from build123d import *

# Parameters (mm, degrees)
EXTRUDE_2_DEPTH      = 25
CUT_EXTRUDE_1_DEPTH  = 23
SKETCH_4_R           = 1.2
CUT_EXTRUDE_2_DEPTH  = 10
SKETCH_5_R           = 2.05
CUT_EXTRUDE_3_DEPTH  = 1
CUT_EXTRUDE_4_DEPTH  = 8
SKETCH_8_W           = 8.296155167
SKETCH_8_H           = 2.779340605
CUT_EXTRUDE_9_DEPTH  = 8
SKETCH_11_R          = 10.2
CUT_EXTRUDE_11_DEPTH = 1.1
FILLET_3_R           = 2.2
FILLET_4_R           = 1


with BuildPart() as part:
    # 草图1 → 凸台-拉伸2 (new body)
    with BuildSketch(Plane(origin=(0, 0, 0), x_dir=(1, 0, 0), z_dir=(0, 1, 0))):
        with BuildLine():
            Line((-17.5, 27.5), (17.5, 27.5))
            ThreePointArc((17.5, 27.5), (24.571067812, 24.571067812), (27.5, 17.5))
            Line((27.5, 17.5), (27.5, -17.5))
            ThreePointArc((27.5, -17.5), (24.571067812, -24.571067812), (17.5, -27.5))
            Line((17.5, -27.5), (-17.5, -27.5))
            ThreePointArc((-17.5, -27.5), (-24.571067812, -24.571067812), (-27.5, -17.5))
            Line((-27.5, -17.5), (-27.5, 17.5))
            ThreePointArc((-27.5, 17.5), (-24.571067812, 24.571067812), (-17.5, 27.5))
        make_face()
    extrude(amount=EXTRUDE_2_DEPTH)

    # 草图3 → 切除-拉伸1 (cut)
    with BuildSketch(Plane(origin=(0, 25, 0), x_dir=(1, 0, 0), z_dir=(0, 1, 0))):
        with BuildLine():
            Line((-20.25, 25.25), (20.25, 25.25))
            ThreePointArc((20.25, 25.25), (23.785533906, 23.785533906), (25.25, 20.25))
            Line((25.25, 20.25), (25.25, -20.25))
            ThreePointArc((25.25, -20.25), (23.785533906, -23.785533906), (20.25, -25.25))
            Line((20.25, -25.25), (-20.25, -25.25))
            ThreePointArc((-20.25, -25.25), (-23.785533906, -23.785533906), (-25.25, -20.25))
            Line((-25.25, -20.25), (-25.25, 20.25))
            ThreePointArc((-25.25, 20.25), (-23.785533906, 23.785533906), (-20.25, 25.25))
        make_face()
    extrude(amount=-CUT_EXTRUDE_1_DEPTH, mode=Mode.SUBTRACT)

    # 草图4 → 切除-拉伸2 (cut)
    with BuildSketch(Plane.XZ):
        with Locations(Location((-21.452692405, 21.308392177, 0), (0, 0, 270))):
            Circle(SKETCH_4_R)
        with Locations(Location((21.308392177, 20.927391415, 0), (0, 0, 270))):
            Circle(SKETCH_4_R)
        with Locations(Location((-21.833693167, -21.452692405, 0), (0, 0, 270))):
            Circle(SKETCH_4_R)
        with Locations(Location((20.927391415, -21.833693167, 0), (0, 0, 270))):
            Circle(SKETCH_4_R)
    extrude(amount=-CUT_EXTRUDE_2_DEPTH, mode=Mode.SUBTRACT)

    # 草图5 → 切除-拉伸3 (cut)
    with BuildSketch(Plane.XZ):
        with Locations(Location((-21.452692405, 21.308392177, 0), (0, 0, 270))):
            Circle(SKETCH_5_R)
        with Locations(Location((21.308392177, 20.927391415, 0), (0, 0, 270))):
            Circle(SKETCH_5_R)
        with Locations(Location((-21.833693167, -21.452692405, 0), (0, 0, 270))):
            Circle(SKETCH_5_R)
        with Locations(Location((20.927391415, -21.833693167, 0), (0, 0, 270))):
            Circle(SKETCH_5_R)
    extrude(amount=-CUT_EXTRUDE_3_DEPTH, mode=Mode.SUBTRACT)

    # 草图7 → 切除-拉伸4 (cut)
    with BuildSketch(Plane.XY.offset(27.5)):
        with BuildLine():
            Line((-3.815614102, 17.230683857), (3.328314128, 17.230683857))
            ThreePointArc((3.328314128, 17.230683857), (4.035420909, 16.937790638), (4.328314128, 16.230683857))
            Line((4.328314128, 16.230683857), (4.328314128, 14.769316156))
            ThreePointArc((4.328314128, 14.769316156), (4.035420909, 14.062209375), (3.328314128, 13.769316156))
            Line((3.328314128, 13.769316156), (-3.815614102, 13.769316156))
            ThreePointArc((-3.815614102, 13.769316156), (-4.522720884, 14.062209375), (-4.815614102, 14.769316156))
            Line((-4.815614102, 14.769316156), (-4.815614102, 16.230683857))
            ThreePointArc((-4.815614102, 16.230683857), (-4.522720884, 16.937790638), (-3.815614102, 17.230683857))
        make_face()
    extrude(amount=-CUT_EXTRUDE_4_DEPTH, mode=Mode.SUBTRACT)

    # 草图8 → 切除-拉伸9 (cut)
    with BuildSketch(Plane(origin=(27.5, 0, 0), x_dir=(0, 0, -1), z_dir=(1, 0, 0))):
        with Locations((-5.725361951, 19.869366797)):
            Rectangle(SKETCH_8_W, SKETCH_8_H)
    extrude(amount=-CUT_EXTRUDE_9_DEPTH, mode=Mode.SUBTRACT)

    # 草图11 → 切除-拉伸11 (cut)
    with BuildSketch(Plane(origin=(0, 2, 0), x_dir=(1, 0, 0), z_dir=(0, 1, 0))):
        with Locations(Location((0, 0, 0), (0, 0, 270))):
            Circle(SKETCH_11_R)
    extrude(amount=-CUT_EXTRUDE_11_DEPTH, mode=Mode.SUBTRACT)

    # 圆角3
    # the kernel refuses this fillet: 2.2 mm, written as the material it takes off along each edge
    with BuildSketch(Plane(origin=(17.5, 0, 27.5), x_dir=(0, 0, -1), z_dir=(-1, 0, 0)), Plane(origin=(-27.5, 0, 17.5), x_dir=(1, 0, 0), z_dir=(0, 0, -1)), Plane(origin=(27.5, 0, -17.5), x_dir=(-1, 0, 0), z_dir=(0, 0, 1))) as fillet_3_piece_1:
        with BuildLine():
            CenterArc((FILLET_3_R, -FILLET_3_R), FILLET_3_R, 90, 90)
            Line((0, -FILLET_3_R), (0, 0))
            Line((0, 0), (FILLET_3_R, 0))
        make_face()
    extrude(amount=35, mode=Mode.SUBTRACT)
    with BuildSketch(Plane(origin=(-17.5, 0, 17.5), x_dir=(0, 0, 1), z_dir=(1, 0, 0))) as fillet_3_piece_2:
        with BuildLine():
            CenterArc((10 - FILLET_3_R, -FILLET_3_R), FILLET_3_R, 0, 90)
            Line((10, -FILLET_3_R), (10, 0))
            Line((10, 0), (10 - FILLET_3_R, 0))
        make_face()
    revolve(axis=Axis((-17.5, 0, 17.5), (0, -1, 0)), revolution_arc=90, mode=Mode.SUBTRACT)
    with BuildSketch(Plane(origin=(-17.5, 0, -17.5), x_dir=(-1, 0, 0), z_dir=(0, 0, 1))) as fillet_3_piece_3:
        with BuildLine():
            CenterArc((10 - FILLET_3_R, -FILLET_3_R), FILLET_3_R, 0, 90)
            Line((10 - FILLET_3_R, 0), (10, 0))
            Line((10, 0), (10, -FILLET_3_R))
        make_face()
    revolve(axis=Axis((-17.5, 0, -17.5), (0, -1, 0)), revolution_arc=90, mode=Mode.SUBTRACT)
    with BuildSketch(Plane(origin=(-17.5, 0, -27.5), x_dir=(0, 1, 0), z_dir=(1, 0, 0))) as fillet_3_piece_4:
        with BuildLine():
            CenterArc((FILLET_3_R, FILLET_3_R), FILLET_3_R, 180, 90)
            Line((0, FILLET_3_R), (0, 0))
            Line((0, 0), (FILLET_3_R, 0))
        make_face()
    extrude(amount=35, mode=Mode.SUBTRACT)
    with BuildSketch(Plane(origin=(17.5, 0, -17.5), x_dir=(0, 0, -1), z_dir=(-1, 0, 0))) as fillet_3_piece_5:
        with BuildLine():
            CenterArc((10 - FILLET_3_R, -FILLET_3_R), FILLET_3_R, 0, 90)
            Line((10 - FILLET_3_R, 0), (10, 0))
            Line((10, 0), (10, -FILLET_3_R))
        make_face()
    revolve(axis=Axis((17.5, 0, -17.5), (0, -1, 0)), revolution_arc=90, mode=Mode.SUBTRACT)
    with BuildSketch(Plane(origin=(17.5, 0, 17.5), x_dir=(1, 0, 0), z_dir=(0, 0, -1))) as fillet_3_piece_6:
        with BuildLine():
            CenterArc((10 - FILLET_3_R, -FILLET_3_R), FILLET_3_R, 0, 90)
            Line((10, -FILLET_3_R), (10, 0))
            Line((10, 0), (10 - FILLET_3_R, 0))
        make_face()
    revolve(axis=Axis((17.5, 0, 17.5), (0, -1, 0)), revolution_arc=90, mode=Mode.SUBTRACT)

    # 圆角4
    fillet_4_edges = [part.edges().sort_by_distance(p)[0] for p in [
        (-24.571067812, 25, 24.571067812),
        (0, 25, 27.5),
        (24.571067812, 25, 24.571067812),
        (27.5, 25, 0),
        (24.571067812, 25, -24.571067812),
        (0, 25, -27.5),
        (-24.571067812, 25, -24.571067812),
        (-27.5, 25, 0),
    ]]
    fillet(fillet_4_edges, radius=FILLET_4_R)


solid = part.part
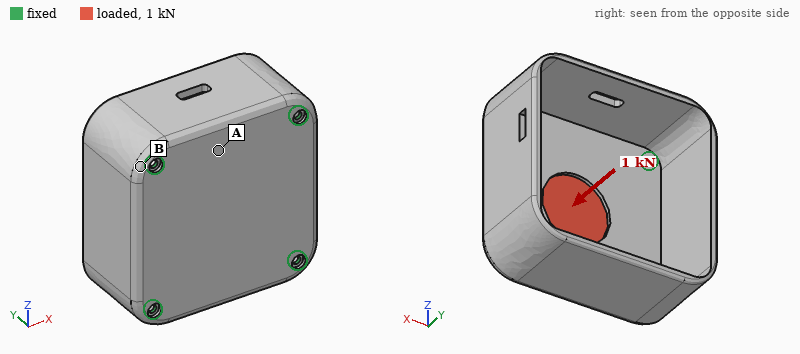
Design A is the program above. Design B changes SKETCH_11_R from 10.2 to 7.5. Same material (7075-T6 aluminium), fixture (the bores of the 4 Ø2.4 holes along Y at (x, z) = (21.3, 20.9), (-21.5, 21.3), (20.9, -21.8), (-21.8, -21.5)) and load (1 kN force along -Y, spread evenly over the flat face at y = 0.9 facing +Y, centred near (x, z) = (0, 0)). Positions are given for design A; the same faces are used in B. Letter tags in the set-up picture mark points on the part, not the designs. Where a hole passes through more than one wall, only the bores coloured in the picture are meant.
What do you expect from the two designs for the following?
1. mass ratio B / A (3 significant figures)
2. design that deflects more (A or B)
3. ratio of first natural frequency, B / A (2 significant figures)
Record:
1.01
A
1.0
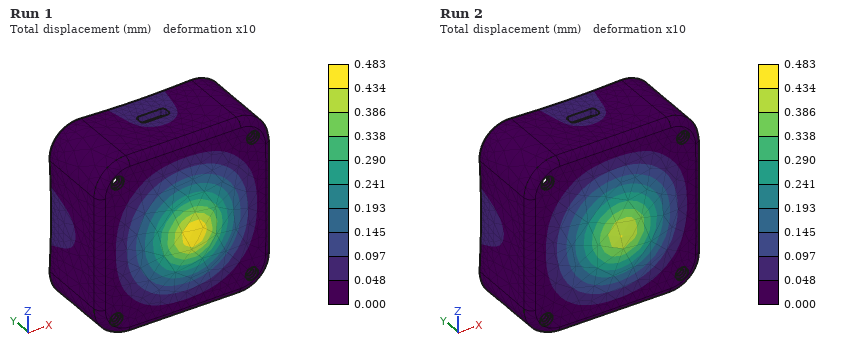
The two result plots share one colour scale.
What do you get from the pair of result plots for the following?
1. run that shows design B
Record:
Run 2
